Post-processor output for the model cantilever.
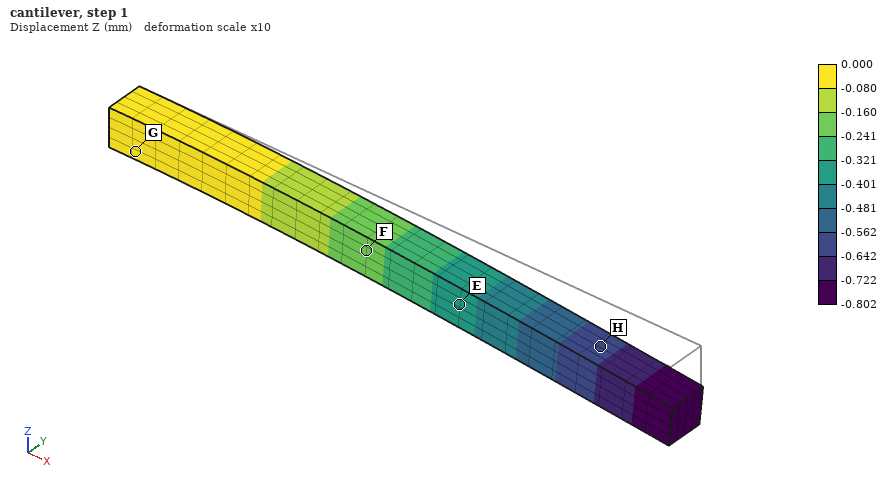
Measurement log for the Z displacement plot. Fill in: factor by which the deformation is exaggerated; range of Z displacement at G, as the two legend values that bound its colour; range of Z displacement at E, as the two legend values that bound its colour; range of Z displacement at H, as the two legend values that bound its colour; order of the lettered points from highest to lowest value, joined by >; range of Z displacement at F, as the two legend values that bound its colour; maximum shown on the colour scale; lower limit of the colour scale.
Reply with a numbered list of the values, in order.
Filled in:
1. 10
2. -0.080 to 0.000 mm
3. -0.401 to -0.321 mm
4. -0.642 to -0.562 mm
5. G > F > E > H
6. -0.241 to -0.160 mm
7. 0.000 mm
8. -0.802 mm
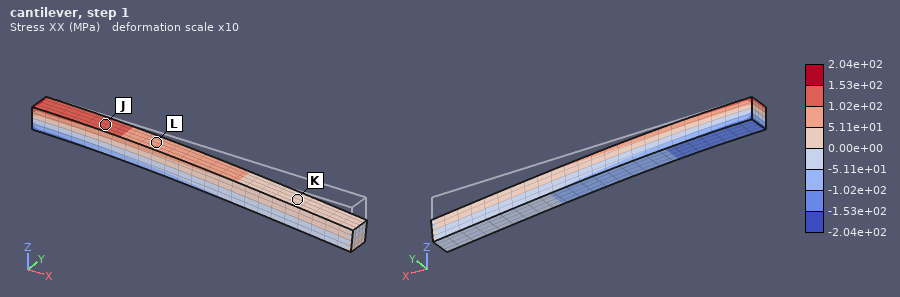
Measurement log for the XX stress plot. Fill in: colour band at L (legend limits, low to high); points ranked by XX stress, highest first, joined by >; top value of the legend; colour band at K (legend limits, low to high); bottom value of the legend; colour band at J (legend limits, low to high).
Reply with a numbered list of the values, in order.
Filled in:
1. 5.11e+01 to 1.02e+02 MPa
2. J > L > K
3. 2.04e+02 MPa
4. 0.00e+00 to 5.11e+01 MPa
5. -2.04e+02 MPa
6. 1.02e+02 to 1.53e+02 MPa
